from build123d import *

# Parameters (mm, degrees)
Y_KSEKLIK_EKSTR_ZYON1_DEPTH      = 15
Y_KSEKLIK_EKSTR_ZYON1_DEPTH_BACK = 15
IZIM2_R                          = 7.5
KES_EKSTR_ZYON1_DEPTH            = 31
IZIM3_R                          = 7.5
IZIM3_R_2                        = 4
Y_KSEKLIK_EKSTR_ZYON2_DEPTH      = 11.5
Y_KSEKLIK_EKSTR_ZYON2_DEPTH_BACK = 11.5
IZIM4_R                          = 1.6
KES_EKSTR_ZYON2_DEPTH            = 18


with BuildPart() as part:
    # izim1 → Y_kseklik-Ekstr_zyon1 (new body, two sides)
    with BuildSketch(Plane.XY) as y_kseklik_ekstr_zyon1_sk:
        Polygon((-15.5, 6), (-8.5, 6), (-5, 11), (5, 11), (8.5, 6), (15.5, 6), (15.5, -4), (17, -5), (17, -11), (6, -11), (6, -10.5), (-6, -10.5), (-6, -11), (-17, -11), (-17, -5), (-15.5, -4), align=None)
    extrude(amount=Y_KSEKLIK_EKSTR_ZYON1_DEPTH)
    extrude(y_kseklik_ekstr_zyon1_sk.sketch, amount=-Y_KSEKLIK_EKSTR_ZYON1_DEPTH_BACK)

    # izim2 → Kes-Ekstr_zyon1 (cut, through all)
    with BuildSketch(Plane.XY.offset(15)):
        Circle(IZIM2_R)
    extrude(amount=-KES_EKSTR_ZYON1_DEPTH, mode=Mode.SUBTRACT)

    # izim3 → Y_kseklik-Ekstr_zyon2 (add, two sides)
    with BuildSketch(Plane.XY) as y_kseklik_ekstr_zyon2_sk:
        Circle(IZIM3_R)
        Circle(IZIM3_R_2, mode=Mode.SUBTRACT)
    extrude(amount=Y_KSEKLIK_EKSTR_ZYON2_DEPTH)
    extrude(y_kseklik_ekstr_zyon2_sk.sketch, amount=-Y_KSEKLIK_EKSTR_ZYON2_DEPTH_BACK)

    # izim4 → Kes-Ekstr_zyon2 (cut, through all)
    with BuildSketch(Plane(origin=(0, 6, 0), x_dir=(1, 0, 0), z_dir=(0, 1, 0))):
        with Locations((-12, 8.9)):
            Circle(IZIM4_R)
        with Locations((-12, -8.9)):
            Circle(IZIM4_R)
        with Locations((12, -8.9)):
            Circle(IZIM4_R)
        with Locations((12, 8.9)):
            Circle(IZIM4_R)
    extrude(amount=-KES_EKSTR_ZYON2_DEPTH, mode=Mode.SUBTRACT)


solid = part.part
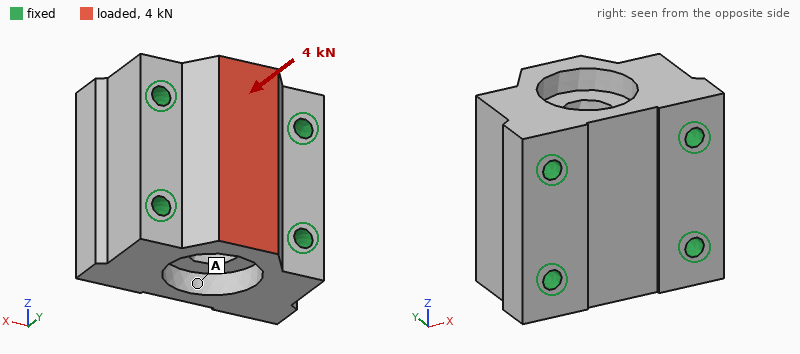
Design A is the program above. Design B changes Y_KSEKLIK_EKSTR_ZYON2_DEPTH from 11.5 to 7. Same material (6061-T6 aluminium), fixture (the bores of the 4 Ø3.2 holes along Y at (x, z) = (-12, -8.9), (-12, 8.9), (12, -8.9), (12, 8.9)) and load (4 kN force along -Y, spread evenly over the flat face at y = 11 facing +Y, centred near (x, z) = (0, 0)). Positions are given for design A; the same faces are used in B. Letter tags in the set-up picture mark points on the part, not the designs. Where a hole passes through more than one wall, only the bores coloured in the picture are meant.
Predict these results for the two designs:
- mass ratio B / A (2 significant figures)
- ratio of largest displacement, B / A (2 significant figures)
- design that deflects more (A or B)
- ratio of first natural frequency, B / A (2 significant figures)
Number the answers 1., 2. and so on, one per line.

1. 0.96
2. 1.3
3. B
4. 1.00
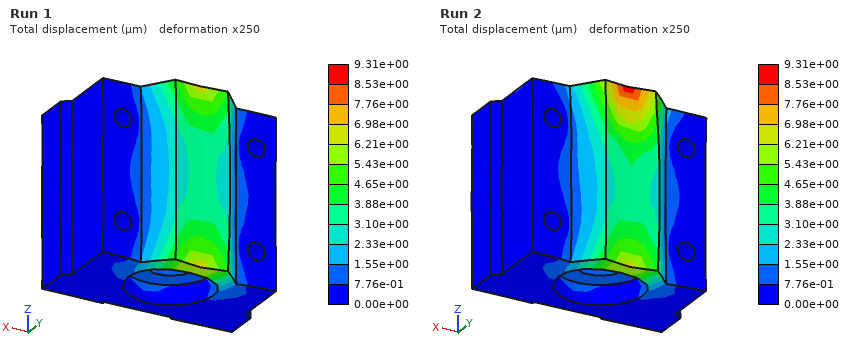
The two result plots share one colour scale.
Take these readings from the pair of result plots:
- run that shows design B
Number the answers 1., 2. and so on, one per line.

1. Run 2
